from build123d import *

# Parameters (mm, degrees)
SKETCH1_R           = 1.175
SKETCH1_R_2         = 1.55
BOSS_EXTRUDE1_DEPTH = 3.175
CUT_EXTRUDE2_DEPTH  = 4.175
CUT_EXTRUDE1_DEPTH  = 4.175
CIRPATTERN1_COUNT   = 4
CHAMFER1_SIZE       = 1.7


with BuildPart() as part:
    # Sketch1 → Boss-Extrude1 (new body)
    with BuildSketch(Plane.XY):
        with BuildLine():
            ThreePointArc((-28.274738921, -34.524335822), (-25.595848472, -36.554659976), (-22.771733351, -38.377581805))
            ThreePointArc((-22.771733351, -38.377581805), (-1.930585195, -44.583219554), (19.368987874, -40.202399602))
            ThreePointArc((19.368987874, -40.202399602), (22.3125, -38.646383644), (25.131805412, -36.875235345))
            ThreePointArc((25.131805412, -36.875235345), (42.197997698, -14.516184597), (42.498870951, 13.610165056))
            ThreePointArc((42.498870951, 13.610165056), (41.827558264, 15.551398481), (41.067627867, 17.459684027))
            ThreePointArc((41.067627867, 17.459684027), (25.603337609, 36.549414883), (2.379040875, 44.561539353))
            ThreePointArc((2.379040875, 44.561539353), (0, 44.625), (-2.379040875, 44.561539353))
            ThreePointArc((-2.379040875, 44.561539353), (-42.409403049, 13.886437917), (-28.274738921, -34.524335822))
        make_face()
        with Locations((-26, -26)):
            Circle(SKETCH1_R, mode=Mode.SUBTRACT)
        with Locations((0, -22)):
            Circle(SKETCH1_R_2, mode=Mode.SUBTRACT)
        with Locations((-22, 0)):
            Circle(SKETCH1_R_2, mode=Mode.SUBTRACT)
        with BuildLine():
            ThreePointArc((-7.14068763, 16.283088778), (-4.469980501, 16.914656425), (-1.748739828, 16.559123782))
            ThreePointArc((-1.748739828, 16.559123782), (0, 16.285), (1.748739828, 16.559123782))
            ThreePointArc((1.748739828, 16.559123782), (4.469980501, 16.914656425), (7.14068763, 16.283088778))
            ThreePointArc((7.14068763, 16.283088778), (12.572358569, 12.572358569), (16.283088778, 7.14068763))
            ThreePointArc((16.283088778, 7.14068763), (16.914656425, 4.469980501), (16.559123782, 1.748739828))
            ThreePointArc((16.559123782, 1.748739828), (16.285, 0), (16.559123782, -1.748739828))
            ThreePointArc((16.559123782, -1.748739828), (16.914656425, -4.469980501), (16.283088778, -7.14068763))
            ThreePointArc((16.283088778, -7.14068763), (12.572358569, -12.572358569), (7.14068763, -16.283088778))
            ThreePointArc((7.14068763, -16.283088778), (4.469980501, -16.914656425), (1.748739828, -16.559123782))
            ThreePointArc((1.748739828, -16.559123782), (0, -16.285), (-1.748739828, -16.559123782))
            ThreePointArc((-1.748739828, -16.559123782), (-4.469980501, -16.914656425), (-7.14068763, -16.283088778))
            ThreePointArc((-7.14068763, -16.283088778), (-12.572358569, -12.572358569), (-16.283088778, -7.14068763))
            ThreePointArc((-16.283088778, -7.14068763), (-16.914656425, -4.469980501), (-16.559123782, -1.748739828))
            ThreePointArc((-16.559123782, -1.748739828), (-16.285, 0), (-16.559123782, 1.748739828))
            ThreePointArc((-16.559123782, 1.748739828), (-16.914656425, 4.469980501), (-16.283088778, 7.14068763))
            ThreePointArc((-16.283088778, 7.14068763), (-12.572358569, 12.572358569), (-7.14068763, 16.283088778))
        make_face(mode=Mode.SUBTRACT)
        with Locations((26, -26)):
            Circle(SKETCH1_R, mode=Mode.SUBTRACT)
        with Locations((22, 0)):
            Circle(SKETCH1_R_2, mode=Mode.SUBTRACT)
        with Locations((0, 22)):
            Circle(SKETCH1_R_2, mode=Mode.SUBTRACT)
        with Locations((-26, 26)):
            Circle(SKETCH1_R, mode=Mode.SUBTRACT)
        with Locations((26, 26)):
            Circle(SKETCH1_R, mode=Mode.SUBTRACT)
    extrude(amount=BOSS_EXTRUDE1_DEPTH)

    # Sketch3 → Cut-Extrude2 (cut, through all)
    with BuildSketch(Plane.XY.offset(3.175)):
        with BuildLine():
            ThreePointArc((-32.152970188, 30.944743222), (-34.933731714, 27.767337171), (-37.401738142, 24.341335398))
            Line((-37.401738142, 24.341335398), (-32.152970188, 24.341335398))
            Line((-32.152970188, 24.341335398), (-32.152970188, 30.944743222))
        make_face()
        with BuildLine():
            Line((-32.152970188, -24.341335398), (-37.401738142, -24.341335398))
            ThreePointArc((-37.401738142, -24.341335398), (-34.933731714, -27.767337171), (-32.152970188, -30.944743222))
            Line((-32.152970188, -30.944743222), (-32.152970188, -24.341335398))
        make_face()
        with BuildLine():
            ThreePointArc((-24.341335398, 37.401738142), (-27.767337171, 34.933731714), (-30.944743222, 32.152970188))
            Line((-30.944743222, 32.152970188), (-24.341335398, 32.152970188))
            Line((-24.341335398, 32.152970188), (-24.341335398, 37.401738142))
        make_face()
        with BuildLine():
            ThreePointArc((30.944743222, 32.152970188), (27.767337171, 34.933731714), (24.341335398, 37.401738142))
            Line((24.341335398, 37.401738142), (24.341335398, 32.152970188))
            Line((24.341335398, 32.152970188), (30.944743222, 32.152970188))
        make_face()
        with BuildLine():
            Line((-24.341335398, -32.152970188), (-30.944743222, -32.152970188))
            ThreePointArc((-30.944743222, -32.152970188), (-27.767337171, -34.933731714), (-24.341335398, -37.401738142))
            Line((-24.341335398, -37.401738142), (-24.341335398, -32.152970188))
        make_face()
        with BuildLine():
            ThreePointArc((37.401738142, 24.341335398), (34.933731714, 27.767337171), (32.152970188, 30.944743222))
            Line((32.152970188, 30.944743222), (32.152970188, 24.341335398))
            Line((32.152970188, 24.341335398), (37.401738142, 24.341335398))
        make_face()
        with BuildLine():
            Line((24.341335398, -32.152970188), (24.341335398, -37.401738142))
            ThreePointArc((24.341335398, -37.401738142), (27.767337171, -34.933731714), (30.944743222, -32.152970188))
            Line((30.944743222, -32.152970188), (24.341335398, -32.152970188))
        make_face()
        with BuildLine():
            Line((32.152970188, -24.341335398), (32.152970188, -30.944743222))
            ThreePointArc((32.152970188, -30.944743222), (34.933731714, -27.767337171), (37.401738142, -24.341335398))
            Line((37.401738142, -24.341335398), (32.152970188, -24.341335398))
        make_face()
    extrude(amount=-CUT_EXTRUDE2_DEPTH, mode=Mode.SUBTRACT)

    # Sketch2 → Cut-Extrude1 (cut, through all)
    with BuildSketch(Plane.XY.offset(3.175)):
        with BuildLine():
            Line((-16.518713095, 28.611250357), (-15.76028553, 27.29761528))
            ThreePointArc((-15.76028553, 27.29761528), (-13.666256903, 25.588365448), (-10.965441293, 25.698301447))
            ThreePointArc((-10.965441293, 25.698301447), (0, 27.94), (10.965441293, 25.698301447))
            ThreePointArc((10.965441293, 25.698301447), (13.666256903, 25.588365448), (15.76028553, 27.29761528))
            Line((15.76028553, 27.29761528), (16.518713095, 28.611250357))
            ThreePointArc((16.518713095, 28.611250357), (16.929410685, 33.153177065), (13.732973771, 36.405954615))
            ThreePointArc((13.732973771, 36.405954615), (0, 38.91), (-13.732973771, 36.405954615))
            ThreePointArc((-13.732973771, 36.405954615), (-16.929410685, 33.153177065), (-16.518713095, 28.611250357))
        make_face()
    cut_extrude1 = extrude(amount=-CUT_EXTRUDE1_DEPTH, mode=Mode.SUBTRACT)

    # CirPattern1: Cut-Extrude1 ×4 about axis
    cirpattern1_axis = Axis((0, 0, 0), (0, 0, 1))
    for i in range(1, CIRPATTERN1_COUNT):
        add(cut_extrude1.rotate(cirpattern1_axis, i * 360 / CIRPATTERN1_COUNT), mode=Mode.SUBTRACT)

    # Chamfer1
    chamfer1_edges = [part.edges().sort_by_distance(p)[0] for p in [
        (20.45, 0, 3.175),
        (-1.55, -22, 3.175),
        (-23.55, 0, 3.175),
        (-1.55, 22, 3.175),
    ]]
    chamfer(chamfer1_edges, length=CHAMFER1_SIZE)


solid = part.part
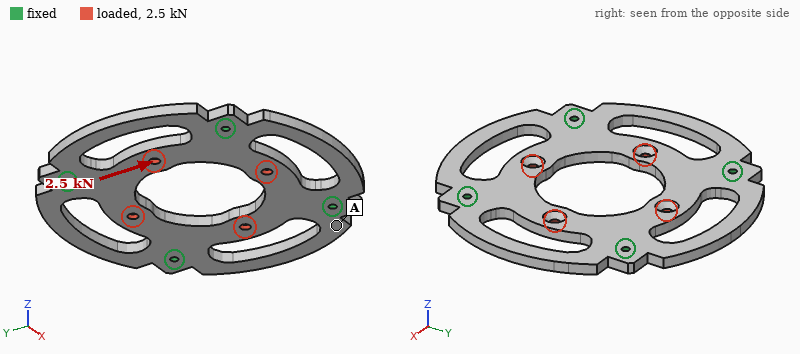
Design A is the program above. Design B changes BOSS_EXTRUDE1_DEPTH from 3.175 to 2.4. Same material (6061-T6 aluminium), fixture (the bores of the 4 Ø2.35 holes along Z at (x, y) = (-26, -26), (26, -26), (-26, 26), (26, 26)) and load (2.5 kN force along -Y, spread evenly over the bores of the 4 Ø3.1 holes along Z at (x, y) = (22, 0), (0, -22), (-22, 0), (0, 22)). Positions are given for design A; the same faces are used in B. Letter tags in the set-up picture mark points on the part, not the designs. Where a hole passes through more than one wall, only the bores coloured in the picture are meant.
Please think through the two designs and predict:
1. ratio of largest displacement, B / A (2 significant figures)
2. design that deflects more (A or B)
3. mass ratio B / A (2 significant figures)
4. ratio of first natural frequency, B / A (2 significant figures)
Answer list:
1.6
B
0.75
0.78
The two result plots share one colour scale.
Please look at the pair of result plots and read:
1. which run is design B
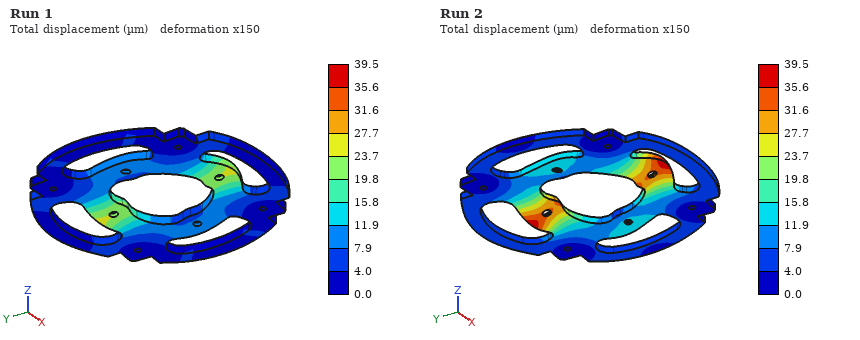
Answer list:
Run 2
